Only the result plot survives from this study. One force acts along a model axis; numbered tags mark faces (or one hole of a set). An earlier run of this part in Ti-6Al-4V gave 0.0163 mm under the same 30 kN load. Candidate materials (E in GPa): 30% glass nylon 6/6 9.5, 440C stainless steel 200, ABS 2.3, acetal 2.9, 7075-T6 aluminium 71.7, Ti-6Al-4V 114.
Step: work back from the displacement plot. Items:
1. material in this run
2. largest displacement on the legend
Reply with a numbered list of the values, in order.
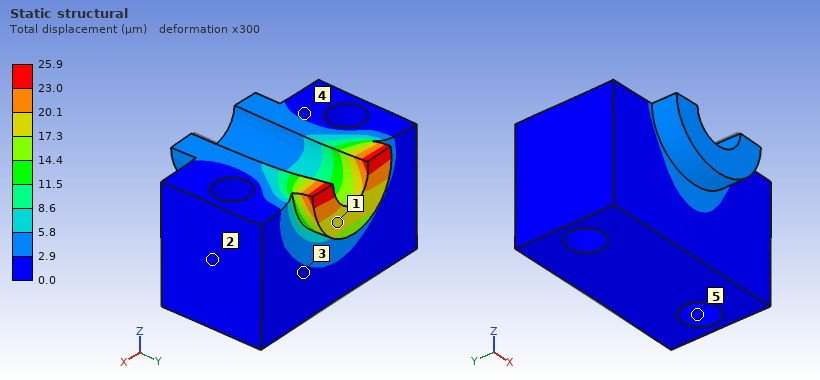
1. 7075-T6 aluminium
2. 25.9 µm
